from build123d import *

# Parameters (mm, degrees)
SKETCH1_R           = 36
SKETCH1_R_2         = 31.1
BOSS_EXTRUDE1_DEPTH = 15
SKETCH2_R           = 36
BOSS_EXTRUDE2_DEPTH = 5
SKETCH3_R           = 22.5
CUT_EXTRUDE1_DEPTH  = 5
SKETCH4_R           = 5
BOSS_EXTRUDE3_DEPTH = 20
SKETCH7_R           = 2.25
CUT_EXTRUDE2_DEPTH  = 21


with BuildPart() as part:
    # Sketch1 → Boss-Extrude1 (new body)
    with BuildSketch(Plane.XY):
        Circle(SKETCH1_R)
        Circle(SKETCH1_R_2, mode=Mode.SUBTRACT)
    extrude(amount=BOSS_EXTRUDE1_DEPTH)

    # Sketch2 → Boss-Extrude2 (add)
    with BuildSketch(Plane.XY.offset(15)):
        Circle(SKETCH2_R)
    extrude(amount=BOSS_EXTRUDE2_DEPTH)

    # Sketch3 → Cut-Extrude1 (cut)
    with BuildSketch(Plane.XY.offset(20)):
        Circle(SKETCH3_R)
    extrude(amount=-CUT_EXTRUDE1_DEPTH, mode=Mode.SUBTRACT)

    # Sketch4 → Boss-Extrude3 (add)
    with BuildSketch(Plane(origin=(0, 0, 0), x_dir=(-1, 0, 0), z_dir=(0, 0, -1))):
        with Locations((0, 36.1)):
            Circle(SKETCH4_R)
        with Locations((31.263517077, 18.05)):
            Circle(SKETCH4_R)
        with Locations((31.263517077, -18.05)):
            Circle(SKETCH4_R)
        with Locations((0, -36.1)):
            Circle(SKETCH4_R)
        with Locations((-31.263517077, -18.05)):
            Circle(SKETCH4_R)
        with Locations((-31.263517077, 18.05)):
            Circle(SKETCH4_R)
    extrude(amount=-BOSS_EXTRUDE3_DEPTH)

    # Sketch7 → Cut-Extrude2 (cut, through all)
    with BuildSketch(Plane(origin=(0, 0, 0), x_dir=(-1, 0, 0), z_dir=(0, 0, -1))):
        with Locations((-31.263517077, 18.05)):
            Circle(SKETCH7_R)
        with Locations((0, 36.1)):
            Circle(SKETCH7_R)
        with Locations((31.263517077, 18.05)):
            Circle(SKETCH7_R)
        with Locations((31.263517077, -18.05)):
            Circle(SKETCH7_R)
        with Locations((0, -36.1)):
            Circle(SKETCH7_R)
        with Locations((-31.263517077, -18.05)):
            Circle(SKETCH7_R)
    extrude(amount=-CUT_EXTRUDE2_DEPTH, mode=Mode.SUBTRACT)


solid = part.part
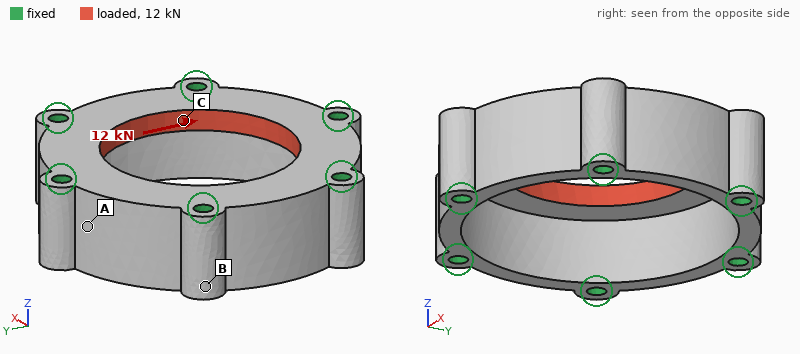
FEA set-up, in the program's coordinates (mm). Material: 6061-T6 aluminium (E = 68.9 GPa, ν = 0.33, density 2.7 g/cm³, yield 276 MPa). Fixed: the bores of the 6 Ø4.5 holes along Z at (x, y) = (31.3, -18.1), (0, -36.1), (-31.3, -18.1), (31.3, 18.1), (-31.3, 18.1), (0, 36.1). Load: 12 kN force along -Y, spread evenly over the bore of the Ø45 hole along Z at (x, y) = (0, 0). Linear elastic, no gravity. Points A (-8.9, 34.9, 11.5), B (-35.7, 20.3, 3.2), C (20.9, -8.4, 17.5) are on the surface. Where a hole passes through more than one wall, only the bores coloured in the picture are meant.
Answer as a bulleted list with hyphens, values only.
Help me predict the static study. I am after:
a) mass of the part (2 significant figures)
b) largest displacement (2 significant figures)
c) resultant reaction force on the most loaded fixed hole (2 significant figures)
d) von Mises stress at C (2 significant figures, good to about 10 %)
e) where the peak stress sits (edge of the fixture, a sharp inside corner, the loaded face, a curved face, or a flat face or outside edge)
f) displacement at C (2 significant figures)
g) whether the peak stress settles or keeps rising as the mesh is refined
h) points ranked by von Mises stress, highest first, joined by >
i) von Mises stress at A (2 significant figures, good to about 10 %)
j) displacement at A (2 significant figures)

- 84 g
- 11 µm
- 2.5 kN
- 32 MPa
- edge of the fixture
- 6.8 µm
- keeps rising
- C > A > B
- 10 MPa
- 2.6 µm
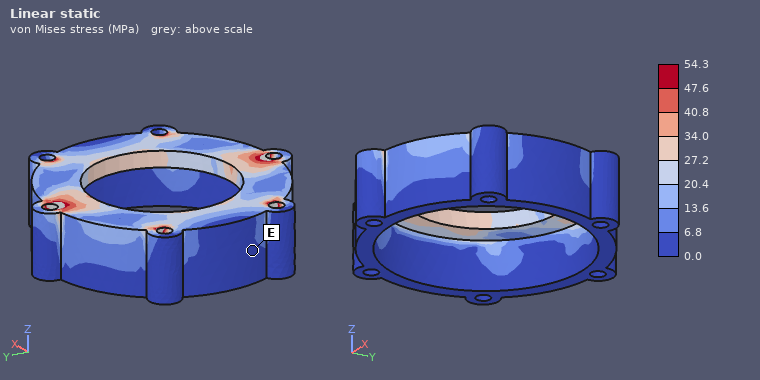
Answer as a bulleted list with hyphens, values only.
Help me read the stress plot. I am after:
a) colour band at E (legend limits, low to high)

- 0.0 to 6.8 MPa
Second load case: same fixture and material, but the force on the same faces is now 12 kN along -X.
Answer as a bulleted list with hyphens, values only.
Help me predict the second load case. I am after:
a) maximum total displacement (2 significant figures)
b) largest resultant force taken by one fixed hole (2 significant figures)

- 13 µm
- 2.3 kN
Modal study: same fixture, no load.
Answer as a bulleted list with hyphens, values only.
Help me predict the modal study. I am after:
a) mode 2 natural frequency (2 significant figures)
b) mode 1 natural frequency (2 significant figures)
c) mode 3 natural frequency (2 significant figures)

- 27 kHz
- 26 kHz
- 27 kHz
